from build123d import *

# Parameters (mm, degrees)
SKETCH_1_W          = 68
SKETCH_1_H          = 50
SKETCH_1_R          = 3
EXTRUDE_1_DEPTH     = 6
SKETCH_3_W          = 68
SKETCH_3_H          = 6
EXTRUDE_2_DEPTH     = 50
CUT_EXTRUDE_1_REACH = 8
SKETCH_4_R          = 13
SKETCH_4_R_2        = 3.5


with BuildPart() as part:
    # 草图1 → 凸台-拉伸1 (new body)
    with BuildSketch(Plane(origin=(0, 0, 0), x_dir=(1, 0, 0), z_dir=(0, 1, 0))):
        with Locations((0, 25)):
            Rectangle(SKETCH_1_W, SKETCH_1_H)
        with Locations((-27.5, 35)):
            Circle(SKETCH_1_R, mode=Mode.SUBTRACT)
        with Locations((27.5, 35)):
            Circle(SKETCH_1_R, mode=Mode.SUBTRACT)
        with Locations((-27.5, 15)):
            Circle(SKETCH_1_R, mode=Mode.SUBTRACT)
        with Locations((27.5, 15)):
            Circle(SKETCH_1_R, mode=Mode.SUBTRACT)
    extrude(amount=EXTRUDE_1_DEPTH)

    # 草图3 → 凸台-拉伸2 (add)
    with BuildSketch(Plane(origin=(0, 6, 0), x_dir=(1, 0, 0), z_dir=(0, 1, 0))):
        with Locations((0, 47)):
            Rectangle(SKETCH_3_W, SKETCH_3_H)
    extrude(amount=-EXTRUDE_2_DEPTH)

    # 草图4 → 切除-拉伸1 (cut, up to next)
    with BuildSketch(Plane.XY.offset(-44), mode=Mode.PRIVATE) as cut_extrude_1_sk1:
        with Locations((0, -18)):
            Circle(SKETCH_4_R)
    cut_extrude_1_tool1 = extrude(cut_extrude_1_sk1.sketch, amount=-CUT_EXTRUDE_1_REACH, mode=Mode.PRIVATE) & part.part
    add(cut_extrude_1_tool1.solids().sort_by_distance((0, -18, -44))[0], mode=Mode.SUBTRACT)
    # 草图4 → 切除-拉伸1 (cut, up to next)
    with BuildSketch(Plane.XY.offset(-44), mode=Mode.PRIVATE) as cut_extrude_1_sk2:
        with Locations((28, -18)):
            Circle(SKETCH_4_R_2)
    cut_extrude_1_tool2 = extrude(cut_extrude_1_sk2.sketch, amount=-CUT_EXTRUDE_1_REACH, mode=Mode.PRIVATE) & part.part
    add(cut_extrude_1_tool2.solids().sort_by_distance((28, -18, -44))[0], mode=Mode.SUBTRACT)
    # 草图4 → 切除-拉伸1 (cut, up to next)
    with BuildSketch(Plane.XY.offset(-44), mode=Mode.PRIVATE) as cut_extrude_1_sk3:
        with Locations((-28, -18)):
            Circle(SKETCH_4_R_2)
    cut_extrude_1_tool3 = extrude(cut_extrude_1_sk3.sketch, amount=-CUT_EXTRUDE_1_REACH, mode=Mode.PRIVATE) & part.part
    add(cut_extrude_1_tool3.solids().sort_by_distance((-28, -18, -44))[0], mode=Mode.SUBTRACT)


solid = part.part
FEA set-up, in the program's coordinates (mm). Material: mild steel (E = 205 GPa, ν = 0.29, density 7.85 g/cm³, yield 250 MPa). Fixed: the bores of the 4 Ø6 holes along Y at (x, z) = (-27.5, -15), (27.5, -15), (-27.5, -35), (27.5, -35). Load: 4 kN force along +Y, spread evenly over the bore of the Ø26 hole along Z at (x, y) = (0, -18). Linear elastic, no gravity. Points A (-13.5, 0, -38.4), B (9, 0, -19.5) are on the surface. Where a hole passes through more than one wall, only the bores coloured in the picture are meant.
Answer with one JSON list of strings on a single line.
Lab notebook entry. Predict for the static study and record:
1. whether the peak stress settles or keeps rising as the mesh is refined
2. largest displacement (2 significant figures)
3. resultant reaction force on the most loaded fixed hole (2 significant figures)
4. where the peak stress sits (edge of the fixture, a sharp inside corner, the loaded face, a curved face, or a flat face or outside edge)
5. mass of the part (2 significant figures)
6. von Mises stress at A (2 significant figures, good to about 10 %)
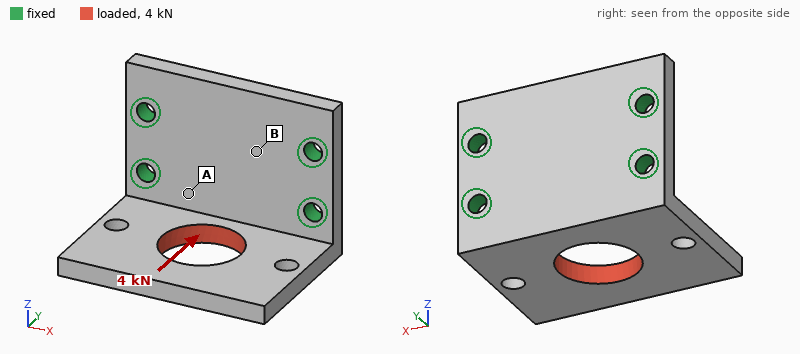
["keeps rising", "67 µm", "2.3 kN", "edge of the fixture", "270 g", "39 MPa"]
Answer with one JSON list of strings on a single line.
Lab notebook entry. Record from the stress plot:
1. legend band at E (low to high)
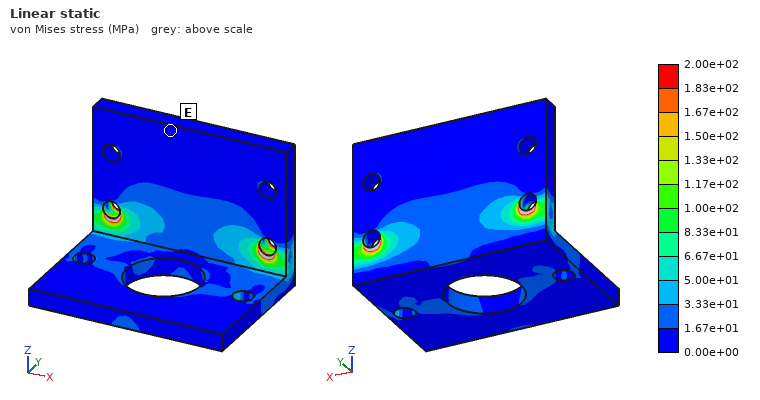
["0.00e+00 to 1.67e+01 MPa"]
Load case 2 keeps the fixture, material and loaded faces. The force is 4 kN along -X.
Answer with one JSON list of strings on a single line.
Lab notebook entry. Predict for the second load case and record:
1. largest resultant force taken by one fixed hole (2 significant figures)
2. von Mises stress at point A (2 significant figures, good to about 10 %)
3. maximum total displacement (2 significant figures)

["2.4 kN", "34 MPa", "33 µm"]
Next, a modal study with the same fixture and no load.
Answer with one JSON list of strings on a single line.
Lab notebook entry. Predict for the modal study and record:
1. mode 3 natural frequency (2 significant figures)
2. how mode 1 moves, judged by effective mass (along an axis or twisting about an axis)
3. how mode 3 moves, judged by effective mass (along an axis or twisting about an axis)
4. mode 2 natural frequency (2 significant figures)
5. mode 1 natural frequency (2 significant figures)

["6000 Hz", "along Z", "along X", "3200 Hz", "1500 Hz"]
